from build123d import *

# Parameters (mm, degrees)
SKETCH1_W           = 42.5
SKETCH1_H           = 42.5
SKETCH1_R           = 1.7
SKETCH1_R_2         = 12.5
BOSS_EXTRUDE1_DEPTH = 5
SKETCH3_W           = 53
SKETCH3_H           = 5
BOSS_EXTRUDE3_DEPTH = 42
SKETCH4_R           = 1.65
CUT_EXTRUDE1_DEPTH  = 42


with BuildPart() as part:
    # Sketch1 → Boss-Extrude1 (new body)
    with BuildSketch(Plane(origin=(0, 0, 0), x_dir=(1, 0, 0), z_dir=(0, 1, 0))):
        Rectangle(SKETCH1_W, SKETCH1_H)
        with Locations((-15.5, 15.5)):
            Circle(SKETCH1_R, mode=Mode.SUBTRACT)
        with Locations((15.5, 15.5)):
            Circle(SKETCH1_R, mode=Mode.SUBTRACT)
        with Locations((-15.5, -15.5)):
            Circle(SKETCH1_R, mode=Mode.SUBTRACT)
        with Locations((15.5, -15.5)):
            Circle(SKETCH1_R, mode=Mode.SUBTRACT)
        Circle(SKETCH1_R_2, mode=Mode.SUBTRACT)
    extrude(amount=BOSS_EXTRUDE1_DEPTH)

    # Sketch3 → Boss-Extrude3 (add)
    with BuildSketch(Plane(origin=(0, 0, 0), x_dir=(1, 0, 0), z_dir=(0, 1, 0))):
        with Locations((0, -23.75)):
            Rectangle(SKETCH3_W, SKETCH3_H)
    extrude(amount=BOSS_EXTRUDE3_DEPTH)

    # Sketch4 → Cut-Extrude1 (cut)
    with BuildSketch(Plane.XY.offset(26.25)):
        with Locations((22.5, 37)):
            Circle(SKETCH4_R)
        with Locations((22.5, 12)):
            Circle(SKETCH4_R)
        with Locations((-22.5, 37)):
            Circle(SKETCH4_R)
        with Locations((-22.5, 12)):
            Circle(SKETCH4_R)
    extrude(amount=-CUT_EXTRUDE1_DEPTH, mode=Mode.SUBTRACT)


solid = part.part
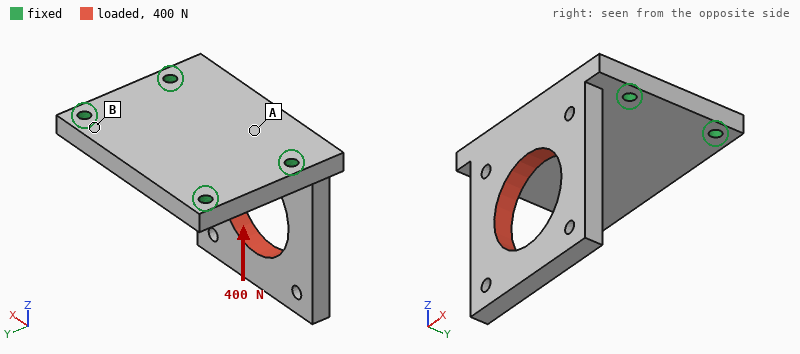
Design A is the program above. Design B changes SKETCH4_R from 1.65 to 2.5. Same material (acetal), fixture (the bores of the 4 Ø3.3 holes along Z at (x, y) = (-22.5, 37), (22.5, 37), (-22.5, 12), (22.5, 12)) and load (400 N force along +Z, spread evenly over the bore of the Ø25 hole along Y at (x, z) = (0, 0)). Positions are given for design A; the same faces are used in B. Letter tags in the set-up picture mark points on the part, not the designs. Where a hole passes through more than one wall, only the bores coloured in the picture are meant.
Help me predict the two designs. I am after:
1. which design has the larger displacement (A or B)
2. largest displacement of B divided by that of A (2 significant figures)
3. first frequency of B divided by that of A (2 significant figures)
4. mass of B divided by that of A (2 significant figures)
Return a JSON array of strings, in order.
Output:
["A", "0.81", "1.0", "0.99"]
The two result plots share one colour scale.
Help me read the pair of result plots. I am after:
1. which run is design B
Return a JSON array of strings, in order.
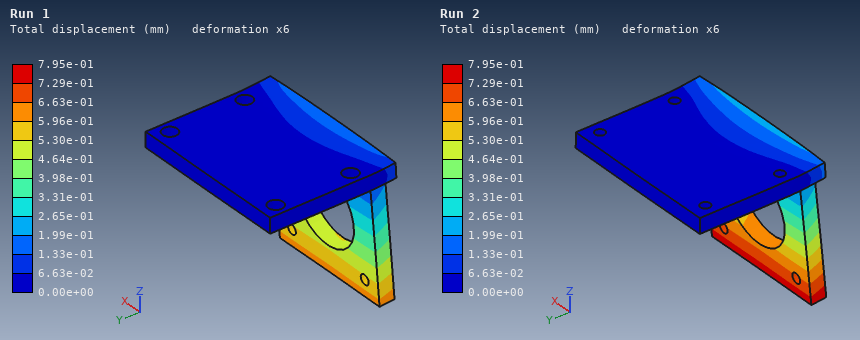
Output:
["Run 1"]
